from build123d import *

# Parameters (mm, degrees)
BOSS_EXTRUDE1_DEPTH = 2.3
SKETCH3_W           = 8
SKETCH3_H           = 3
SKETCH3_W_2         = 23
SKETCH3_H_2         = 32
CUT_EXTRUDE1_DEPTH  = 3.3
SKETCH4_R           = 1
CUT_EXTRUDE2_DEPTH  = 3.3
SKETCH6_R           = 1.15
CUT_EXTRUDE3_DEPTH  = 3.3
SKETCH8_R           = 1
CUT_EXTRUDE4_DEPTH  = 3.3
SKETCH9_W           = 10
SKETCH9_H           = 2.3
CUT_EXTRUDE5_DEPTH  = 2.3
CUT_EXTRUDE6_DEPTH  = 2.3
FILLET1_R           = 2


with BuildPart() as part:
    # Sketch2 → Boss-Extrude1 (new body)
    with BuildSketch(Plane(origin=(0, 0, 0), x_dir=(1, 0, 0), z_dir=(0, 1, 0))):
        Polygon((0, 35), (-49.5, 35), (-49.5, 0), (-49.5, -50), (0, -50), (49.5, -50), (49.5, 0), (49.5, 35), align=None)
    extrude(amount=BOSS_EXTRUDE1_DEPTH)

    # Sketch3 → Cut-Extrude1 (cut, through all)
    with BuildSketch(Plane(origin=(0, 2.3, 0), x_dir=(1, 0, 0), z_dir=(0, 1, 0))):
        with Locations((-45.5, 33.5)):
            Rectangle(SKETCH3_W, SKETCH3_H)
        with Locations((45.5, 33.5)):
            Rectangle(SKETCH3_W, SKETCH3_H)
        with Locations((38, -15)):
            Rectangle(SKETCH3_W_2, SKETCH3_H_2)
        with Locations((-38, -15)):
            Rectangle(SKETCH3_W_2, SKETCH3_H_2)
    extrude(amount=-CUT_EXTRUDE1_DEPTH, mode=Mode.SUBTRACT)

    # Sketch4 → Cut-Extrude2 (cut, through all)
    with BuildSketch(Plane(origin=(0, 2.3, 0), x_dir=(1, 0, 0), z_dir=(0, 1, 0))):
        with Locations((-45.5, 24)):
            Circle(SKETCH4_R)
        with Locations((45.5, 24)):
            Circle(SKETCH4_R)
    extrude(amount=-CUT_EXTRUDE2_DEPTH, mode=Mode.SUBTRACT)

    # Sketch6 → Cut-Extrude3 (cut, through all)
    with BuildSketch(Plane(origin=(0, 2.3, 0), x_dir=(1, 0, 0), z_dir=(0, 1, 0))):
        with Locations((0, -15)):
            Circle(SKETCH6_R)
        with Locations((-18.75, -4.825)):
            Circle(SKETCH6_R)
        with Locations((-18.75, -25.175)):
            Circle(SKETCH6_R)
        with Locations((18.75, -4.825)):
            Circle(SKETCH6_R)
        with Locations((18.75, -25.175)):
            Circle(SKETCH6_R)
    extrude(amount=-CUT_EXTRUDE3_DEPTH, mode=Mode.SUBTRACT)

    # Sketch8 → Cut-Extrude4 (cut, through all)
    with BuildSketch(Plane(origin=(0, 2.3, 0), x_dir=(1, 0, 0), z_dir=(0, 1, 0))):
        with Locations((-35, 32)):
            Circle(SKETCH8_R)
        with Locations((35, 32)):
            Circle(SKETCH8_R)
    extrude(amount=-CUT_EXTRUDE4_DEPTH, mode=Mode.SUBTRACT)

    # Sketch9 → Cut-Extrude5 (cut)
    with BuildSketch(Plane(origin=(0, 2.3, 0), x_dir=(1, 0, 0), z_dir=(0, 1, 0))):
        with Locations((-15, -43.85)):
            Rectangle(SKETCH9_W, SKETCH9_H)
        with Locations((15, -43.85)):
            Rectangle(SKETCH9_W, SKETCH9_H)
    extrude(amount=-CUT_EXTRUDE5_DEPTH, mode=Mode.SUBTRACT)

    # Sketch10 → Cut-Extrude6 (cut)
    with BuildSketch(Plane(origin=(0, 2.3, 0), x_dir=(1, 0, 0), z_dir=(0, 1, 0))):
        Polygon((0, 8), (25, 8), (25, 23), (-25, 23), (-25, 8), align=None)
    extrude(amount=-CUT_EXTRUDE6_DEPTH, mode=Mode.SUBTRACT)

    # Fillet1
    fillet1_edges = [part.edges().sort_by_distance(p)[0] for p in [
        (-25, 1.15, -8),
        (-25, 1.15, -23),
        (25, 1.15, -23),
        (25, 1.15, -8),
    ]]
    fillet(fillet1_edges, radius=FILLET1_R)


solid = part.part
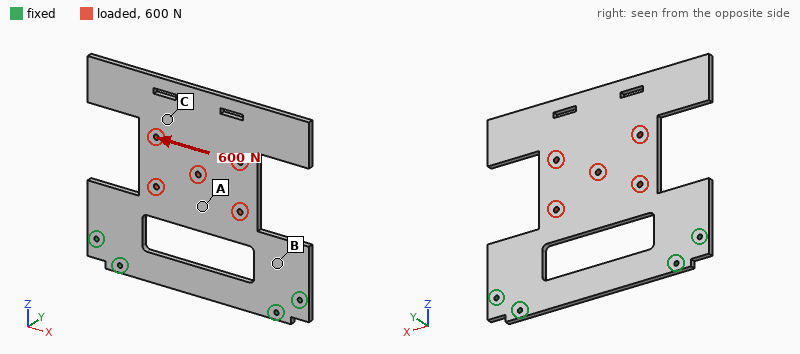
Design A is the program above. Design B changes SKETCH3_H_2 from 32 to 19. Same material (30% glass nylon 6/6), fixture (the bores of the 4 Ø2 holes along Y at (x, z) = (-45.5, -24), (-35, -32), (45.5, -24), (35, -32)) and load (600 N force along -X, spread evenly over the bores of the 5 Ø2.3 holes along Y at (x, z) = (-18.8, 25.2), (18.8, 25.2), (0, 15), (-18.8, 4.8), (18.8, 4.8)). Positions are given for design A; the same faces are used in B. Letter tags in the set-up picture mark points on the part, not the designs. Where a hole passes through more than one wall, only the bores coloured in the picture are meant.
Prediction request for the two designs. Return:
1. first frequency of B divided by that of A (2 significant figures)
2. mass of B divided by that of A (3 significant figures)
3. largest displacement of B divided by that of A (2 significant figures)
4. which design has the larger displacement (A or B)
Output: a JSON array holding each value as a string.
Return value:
["1.1", "1.10", "0.83", "A"]
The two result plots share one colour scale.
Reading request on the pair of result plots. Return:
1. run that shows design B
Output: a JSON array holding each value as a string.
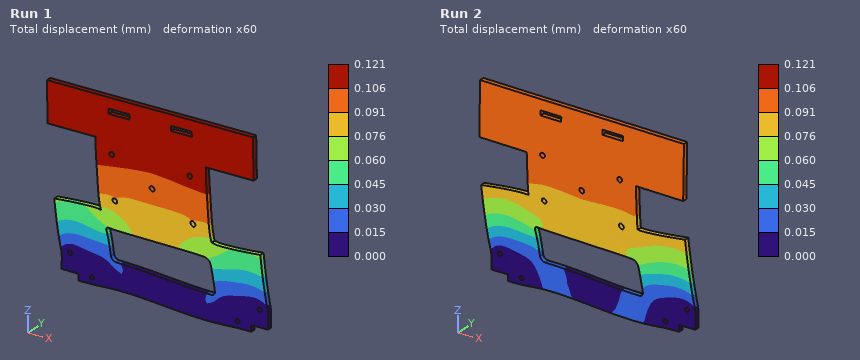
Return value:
["Run 2"]
